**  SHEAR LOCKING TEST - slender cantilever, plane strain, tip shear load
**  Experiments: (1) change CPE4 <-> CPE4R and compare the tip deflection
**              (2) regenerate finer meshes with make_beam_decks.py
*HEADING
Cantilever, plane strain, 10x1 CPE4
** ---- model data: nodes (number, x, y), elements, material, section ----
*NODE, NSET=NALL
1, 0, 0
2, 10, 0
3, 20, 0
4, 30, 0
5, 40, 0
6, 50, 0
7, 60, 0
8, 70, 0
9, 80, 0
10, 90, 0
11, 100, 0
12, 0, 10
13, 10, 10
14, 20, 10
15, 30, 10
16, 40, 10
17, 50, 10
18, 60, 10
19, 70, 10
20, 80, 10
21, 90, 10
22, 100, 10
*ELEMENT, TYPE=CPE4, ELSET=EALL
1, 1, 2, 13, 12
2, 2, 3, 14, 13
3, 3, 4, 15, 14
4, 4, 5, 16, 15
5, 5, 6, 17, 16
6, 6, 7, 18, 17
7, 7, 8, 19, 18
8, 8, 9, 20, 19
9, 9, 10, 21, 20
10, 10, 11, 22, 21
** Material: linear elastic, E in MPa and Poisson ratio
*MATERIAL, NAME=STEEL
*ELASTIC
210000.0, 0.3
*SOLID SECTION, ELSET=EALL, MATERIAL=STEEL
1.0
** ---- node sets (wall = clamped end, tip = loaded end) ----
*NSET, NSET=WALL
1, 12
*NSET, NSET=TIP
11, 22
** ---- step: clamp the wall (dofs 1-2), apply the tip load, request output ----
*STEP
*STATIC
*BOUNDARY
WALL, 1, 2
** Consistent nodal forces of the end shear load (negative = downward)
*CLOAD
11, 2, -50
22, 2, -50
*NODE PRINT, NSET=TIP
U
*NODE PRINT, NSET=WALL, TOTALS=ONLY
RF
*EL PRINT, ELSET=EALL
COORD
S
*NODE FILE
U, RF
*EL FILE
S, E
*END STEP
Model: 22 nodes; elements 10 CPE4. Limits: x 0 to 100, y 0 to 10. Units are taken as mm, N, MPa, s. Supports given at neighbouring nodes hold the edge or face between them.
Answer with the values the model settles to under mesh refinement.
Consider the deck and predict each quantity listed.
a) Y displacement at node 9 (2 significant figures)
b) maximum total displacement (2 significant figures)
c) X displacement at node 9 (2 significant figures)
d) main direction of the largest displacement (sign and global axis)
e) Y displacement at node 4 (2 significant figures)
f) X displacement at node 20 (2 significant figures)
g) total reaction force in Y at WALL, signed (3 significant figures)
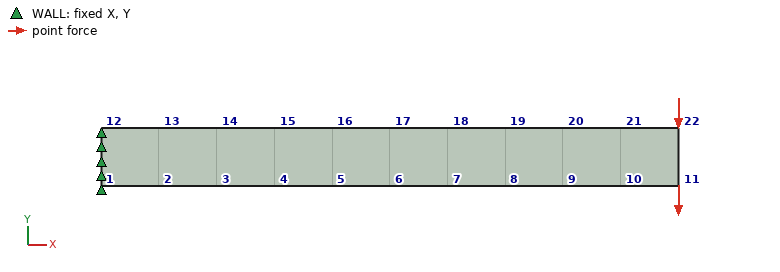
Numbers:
-1.2 mm
1.7 mm
-0.12 mm
-Y
-0.21 mm
0.12 mm
100 N
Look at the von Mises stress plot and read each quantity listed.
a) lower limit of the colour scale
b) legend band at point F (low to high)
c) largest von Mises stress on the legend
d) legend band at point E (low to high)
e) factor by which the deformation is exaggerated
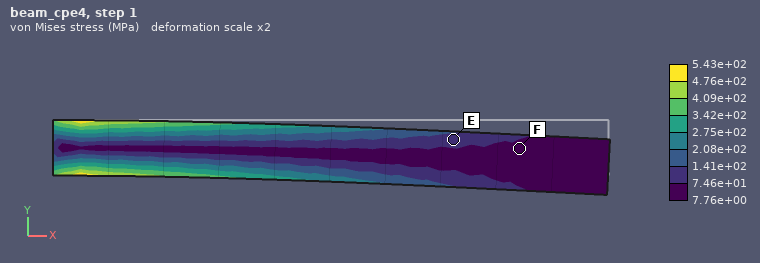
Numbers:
7.76e+00 MPa
7.76e+00 to 7.46e+01 MPa
5.43e+02 MPa
7.46e+01 to 1.41e+02 MPa
2
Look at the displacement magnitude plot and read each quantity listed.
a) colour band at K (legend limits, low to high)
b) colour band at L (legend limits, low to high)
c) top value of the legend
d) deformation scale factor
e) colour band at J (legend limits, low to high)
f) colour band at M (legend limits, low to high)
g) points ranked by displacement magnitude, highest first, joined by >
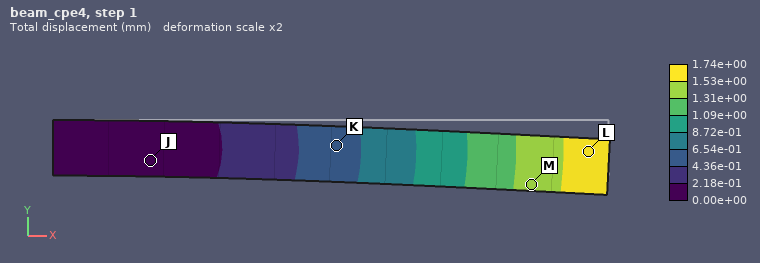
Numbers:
4.36e-01 to 6.54e-01 mm
1.53e+00 to 1.74e+00 mm
1.74e+00 mm
2
0.00e+00 to 2.18e-01 mm
1.31e+00 to 1.53e+00 mm
L > M > K > J
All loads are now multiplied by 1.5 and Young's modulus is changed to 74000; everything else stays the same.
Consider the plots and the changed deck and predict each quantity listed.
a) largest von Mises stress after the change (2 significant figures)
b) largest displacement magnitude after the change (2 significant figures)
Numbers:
810 MPa
7.4 mm
